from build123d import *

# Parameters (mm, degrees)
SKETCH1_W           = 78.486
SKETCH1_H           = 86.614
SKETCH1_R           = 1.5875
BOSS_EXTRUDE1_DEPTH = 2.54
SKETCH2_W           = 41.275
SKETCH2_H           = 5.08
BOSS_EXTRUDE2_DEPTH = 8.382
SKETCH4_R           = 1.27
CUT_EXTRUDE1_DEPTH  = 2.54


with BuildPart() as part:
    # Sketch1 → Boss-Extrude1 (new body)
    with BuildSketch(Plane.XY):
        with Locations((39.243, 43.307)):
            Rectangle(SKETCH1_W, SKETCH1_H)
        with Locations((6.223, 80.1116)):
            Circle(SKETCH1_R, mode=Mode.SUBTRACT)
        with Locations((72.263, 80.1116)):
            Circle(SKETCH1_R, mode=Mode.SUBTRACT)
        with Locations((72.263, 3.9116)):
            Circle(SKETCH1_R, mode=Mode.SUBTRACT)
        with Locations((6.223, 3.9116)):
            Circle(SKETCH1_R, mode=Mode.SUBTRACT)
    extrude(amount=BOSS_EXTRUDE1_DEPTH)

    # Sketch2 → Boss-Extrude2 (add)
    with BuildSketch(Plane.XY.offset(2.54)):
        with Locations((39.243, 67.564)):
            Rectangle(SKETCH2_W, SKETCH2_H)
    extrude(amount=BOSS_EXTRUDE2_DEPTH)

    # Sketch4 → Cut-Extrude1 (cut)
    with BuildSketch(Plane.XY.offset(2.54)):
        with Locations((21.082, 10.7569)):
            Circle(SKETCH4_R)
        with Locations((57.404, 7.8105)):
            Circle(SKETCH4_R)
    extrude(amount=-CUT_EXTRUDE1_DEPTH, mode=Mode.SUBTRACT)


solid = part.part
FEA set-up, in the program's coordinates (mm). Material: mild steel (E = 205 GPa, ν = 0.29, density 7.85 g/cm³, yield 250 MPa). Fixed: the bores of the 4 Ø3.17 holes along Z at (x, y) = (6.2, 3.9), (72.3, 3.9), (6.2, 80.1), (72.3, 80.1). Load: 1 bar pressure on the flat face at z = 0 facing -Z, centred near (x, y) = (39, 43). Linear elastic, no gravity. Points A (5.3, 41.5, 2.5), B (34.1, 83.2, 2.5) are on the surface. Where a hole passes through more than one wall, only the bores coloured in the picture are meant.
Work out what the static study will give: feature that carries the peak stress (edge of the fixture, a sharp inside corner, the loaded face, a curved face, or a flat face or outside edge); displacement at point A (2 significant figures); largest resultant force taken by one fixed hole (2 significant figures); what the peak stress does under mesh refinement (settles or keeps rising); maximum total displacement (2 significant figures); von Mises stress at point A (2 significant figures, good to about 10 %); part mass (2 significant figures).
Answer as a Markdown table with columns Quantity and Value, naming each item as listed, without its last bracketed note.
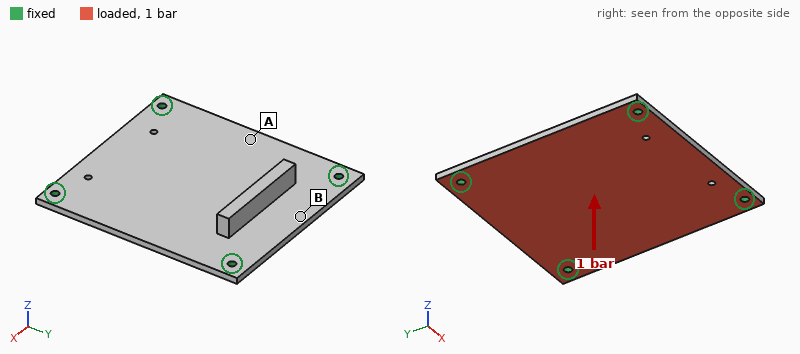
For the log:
| Quantity | Value |
|---|---|
| feature that carries the peak stress | edge of the fixture |
| displacement at point A | 47 µm |
| largest resultant force taken by one fixed hole | 180 N |
| what the peak stress does under mesh refinement | keeps rising |
| maximum total displacement | 60 µm |
| von Mises stress at point A | 30 MPa |
| part mass | 150 g |
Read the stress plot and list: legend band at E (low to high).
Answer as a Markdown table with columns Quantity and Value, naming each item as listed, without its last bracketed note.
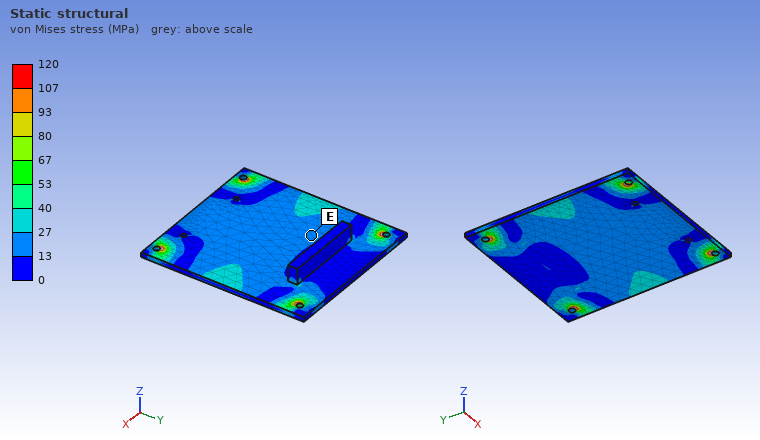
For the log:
| Quantity | Value |
|---|---|
| legend band at E | 13 to 27 MPa |
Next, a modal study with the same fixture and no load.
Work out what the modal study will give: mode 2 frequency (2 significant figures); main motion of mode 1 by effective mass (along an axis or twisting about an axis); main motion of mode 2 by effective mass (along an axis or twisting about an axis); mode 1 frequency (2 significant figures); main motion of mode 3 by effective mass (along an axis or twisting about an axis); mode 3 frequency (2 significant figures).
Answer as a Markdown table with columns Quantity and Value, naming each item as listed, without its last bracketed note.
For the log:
| Quantity | Value |
|---|---|
| mode 2 frequency | 2800 Hz |
| main motion of mode 1 by effective mass | along Z |
| main motion of mode 2 by effective mass | twisting about Y |
| mode 1 frequency | 1700 Hz |
| main motion of mode 3 by effective mass | twisting about X |
| mode 3 frequency | 3100 Hz |
